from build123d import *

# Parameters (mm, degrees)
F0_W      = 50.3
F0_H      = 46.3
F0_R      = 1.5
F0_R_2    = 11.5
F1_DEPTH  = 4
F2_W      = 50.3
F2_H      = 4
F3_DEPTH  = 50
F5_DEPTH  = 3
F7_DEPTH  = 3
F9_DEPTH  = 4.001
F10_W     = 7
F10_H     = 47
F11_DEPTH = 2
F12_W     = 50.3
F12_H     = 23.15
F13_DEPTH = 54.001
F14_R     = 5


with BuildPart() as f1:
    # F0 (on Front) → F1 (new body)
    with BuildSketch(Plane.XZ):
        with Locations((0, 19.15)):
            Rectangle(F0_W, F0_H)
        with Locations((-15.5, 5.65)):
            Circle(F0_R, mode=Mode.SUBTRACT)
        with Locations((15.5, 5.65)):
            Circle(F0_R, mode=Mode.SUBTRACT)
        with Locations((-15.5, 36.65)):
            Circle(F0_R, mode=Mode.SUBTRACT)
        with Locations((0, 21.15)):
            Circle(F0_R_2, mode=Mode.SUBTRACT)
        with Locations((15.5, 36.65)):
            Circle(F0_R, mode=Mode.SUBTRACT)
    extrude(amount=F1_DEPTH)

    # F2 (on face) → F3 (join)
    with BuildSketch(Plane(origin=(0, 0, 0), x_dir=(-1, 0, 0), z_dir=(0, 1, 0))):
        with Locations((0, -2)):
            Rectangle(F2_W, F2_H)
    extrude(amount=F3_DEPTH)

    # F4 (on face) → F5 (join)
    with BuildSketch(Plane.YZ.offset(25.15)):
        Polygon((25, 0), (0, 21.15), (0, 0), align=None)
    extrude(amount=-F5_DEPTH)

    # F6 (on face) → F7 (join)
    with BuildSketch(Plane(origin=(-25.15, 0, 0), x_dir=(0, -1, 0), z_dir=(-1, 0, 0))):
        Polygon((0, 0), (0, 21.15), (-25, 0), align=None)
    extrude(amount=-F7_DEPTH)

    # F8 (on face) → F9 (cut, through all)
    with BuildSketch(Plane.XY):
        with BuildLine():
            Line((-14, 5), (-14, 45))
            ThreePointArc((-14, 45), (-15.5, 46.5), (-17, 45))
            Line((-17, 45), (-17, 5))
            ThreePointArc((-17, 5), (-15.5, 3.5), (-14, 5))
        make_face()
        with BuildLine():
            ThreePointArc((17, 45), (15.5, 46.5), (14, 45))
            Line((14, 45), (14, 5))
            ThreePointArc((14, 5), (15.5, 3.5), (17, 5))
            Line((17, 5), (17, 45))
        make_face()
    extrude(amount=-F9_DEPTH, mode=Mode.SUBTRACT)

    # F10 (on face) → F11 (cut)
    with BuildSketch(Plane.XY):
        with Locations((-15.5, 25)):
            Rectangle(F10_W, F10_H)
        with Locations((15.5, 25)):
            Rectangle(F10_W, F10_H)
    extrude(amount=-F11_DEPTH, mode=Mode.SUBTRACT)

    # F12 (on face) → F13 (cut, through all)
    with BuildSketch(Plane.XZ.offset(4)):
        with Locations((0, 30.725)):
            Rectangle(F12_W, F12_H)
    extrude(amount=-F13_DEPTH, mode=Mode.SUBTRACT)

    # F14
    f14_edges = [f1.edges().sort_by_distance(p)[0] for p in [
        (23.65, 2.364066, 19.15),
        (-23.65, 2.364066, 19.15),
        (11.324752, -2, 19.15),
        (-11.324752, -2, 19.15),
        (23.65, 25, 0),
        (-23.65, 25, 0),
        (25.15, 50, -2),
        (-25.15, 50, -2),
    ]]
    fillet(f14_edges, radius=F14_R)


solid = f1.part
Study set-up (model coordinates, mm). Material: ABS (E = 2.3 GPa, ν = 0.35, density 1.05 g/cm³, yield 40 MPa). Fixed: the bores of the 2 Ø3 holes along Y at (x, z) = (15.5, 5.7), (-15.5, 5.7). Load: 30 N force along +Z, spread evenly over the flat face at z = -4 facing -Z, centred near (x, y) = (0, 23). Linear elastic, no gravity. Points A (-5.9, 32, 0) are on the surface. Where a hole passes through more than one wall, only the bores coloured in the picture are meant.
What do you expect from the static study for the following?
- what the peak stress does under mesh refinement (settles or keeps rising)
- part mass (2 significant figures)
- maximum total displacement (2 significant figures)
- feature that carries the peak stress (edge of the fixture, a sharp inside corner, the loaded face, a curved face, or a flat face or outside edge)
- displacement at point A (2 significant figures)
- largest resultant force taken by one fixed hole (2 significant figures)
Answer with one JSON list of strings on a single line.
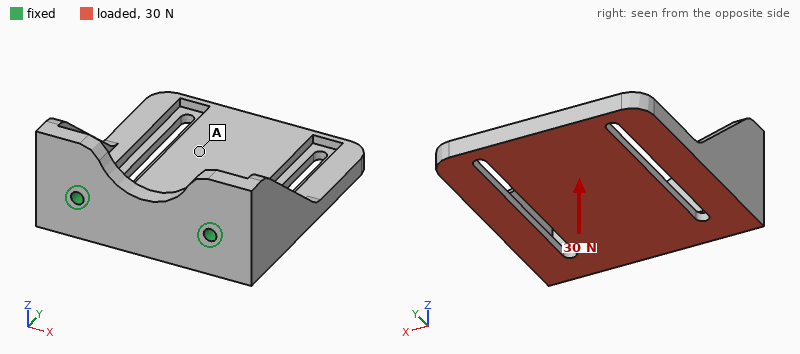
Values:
["keeps rising", "14 g", "0.70 mm", "edge of the fixture", "0.43 mm", "15 N"]
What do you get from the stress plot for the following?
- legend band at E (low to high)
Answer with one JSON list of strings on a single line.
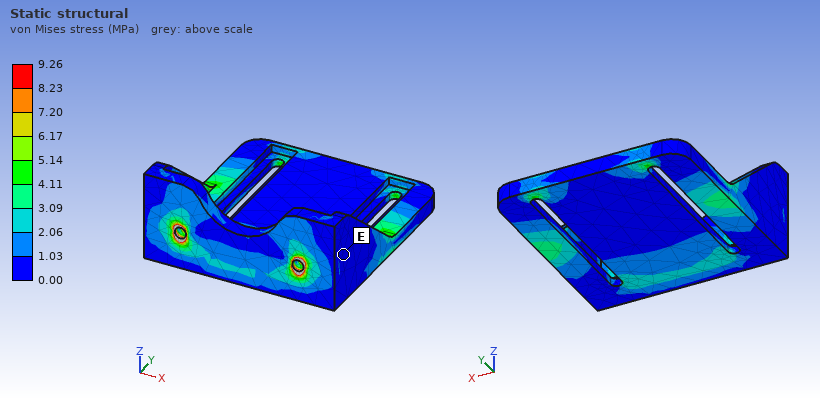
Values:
["0.00 to 1.03 MPa"]
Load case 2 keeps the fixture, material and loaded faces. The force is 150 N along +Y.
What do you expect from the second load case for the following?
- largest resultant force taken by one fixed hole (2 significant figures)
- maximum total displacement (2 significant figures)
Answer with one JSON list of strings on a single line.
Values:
["75 N", "0.77 mm"]
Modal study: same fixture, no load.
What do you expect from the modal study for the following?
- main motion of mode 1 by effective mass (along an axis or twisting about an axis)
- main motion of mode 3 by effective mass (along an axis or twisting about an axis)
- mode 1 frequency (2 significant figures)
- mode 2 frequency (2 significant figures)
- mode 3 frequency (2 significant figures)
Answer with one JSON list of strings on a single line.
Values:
["along Z", "along X", "420 Hz", "890 Hz", "1400 Hz"]
